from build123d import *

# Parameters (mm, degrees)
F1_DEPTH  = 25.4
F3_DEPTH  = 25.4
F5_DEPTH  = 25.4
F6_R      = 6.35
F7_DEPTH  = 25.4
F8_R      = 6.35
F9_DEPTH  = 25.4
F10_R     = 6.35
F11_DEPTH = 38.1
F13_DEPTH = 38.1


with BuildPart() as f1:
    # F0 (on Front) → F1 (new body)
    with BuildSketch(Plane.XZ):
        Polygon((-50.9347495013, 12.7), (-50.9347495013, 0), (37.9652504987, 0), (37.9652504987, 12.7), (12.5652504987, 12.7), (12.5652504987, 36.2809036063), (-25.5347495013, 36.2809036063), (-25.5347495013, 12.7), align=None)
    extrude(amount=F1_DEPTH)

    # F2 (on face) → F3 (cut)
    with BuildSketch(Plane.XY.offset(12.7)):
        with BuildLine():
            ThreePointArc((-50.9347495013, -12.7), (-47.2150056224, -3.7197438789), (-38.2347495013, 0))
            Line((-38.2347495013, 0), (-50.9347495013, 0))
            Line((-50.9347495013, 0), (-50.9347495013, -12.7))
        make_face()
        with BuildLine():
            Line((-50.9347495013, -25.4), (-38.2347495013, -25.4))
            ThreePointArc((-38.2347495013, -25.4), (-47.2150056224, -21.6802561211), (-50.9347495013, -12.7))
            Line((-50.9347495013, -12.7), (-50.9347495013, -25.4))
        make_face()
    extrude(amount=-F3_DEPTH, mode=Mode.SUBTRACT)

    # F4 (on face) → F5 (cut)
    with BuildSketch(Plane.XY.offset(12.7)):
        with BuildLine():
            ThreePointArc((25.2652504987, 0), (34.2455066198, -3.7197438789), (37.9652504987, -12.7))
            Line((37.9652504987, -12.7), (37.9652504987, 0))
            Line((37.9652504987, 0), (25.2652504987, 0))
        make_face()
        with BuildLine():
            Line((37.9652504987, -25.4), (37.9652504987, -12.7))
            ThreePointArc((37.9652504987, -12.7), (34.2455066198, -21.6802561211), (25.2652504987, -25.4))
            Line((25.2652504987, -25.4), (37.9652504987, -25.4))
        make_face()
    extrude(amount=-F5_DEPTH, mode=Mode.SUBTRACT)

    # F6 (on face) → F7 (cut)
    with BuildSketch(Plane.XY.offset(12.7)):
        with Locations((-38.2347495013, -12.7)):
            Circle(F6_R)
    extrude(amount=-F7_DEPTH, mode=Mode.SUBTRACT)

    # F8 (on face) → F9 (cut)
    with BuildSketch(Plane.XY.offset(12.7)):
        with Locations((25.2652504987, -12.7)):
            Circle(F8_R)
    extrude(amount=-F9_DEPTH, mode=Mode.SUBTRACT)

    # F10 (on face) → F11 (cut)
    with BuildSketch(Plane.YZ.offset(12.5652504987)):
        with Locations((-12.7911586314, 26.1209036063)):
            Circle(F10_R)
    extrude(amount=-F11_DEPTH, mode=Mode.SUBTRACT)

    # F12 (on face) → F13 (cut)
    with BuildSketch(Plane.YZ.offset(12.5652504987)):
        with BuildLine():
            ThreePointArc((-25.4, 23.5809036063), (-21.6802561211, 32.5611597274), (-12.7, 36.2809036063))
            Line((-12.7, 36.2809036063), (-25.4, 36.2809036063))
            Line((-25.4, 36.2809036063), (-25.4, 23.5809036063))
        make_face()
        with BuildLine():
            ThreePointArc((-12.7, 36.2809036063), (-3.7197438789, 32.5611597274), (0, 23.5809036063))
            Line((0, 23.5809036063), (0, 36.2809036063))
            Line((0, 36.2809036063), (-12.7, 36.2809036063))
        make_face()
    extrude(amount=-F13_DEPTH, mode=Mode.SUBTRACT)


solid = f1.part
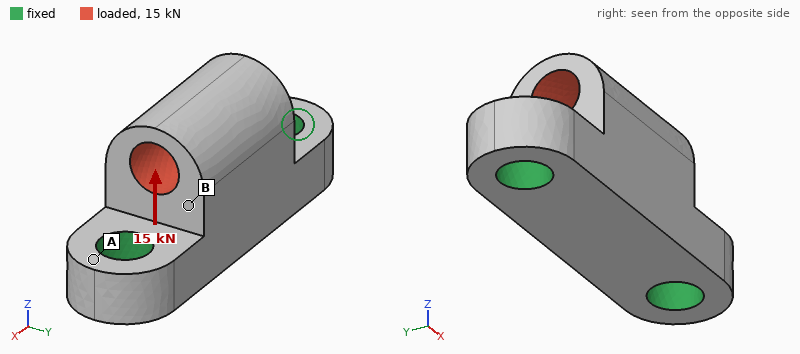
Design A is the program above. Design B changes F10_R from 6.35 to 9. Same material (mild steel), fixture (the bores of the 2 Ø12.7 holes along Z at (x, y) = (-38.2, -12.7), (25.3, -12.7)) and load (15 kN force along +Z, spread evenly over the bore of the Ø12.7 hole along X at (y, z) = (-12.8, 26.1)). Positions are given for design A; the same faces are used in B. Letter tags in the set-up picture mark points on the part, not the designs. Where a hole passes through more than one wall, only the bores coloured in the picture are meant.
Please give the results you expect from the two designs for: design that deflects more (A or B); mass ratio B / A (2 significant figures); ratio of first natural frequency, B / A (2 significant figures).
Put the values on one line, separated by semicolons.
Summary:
B; 0.88; 1.1
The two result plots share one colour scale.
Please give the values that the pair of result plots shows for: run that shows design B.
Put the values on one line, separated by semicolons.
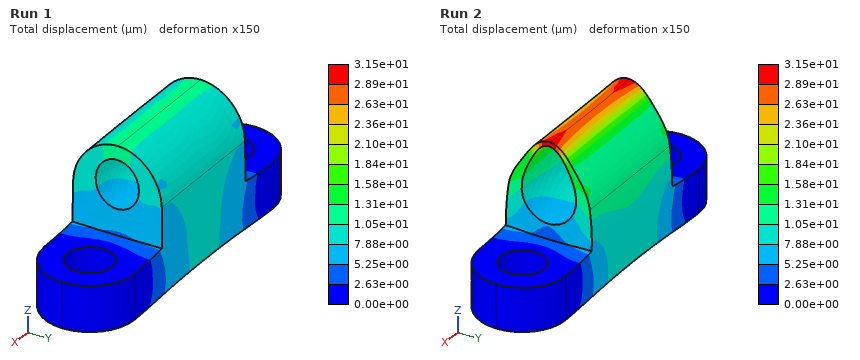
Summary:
Run 2
